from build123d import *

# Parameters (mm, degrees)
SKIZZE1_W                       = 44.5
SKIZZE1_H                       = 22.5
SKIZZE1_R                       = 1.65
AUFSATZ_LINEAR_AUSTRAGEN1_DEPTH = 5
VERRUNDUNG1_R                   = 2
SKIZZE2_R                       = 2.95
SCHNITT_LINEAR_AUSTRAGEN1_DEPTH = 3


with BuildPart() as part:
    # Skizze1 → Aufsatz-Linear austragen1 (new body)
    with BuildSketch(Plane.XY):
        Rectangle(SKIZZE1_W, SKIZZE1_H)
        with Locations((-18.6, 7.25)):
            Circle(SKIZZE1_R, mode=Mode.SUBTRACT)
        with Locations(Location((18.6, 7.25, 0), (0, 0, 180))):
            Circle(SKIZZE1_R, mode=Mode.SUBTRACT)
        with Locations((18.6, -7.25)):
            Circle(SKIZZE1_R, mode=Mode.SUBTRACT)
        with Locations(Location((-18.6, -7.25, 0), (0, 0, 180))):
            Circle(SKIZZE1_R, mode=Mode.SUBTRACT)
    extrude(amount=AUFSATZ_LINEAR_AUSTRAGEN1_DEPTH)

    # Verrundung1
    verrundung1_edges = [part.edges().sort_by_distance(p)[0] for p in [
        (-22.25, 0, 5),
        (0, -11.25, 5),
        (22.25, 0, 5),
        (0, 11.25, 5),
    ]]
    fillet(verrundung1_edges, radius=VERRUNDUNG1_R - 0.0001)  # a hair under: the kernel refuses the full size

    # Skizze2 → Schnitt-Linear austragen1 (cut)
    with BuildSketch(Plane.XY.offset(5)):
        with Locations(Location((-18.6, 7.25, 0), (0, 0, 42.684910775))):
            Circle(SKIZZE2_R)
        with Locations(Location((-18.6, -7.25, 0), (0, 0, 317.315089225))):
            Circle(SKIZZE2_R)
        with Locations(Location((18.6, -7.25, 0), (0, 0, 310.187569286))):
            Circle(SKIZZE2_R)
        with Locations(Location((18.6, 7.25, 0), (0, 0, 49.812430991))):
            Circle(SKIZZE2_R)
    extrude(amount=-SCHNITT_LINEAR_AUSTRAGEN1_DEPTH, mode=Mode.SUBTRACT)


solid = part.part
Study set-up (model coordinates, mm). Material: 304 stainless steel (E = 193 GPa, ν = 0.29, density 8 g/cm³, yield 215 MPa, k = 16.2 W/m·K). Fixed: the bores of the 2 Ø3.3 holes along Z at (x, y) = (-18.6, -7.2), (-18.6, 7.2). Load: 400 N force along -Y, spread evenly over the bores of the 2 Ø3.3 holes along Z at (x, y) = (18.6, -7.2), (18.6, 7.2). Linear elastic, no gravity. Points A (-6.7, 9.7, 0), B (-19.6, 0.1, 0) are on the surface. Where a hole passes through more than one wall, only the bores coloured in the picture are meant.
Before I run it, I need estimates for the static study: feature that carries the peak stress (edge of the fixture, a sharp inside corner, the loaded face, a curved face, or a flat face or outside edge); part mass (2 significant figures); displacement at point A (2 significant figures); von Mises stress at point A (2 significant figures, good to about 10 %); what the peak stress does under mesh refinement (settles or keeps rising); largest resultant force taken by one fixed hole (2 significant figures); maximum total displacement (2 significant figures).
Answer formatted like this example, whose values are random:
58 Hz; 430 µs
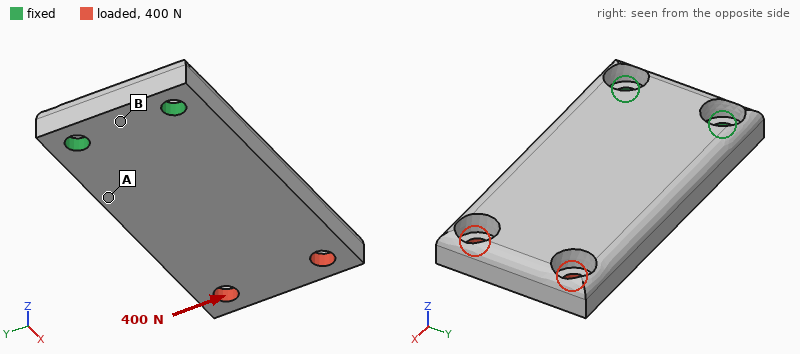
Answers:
edge of the fixture; 36 g; 5.3 µm; 28 MPa; keeps rising; 930 N; 19 µm
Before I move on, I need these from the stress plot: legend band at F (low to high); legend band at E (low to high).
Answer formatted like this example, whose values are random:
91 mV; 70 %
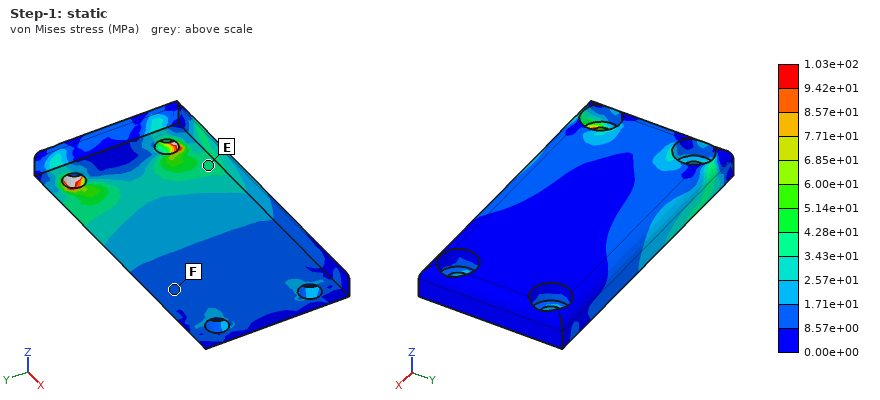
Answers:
8.57e+00 to 1.71e+01 MPa; 3.43e+01 to 4.28e+01 MPa
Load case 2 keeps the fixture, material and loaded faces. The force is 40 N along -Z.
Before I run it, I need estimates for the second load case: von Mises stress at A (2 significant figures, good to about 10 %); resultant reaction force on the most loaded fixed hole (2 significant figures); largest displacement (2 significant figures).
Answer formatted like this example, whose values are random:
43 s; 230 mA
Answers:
11 MPa; 20 N; 33 µm
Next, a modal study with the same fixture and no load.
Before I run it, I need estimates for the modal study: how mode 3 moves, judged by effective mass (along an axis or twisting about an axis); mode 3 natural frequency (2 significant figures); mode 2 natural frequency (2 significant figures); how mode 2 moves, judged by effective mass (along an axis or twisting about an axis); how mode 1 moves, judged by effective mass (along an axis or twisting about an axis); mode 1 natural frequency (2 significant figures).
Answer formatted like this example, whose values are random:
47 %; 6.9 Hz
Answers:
along Y; 9100 Hz; 7400 Hz; along Y; along Z; 1800 Hz
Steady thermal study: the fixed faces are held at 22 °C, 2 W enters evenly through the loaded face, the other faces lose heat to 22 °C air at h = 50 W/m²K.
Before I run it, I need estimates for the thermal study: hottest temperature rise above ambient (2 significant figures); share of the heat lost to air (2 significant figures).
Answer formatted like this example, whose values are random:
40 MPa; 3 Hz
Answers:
28 K; 68 %
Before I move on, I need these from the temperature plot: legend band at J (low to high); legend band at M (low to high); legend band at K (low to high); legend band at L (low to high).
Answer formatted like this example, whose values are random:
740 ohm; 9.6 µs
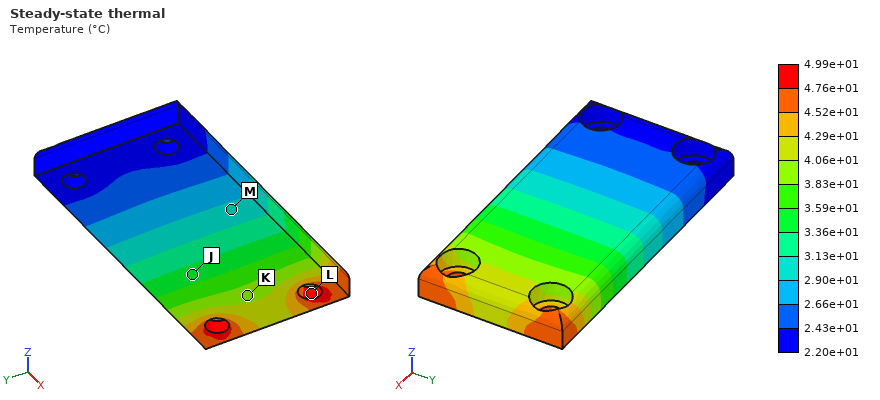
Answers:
3.36e+01 to 3.59e+01 °C; 2.90e+01 to 3.13e+01 °C; 3.83e+01 to 4.06e+01 °C; 4.76e+01 to 4.99e+01 °C
